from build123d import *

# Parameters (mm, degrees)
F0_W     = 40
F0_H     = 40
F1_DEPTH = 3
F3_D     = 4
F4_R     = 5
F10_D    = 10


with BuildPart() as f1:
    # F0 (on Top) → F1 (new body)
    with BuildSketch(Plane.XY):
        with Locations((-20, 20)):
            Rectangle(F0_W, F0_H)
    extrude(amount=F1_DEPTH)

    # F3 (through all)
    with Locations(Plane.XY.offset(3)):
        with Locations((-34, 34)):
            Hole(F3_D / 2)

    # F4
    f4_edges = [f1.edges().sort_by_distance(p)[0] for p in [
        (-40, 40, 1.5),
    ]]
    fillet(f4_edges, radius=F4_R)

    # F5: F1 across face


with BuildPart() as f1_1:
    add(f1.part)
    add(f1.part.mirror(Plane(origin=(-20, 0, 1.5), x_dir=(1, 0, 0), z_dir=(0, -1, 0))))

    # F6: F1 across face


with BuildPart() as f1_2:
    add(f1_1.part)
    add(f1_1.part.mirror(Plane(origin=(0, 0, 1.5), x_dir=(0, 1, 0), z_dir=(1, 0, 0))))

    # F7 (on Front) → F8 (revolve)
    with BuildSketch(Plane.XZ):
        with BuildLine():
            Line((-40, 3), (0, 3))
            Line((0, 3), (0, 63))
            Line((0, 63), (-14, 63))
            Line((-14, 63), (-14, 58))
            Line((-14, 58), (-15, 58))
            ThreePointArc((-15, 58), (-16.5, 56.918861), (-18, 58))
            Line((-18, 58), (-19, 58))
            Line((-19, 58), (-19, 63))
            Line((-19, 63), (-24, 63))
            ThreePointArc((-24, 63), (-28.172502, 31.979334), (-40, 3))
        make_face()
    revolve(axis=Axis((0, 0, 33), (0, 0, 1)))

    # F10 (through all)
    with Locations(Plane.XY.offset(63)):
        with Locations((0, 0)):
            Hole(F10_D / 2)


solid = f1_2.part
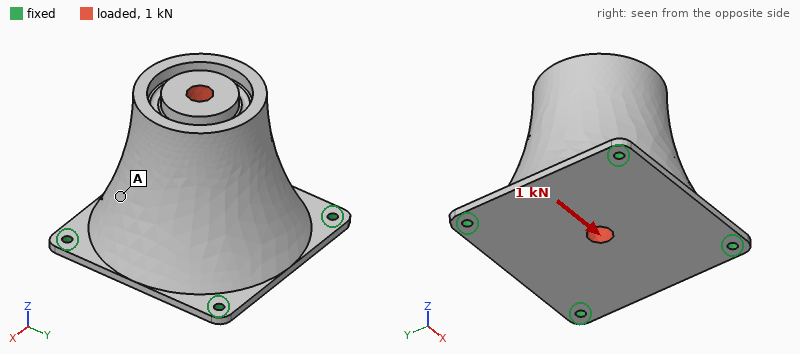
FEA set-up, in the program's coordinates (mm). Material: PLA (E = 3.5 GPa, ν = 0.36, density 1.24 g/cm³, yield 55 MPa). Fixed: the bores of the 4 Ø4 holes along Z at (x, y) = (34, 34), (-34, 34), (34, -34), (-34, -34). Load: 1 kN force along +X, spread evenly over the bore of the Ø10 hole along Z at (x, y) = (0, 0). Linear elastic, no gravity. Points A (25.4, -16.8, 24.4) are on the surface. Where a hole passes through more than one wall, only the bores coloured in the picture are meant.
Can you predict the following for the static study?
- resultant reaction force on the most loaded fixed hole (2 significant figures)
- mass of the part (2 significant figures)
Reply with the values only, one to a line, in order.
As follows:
380 N
220 g
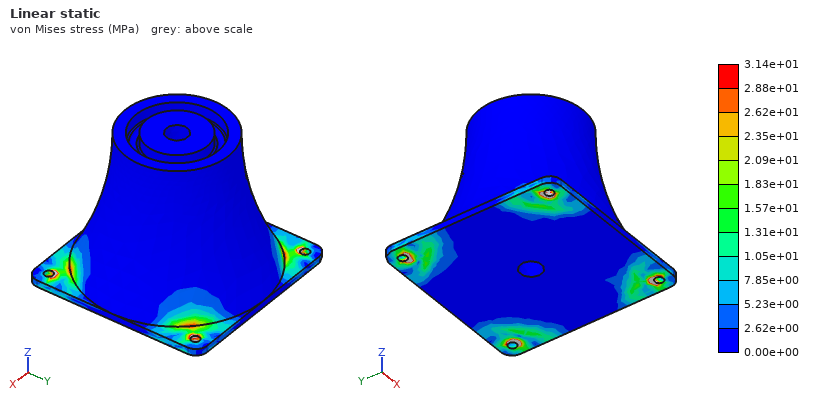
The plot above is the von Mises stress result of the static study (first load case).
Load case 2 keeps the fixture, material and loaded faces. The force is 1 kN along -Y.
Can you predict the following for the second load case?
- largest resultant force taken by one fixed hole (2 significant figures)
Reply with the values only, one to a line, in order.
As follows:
380 N
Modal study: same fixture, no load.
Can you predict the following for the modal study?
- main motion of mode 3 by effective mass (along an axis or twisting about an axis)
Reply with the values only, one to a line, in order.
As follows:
along Z
